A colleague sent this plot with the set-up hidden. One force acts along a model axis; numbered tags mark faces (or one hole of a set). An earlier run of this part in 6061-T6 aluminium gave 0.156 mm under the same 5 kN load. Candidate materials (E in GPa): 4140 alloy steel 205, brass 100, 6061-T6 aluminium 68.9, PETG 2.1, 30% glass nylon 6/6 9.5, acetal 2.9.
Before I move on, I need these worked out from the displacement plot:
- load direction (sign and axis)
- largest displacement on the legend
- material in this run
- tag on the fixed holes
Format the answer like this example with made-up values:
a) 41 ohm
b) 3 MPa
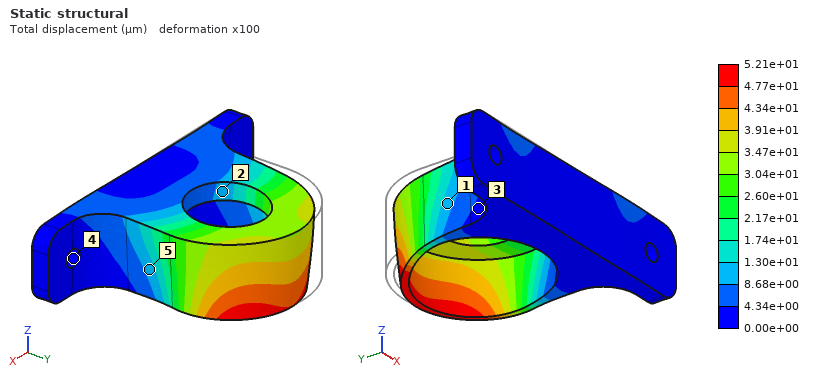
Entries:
a) +X
b) 5.21e+01 µm
c) 4140 alloy steel
d) 4
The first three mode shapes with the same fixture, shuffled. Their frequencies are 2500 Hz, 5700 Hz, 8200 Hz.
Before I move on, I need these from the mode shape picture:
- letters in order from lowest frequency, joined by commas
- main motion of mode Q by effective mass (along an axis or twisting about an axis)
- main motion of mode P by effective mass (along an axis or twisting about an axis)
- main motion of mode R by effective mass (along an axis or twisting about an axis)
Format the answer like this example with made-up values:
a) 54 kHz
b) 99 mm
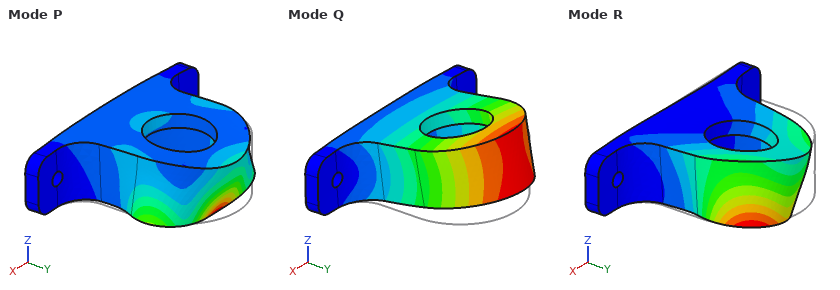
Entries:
a) Q, R, P
b) along Z
c) along Y
d) along X
